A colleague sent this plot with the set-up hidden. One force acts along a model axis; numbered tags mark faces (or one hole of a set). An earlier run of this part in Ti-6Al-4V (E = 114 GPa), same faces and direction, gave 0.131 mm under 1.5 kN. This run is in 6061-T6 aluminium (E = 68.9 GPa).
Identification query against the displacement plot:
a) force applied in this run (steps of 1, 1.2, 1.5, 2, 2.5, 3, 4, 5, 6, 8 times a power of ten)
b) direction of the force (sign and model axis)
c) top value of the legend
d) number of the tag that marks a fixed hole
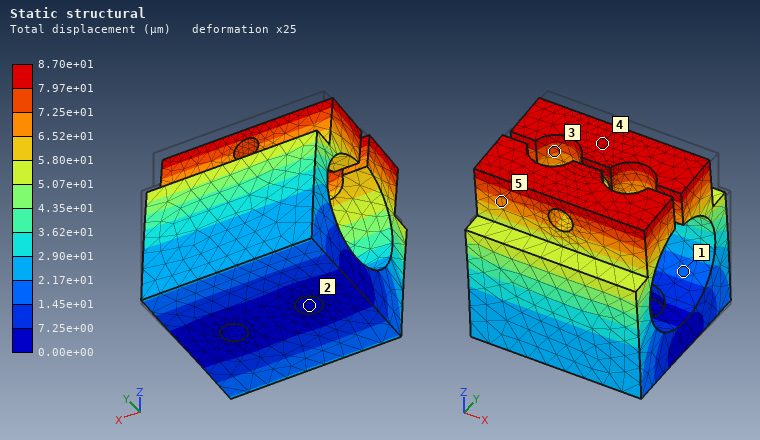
600 N
-Y
8.70e+01 µm
2
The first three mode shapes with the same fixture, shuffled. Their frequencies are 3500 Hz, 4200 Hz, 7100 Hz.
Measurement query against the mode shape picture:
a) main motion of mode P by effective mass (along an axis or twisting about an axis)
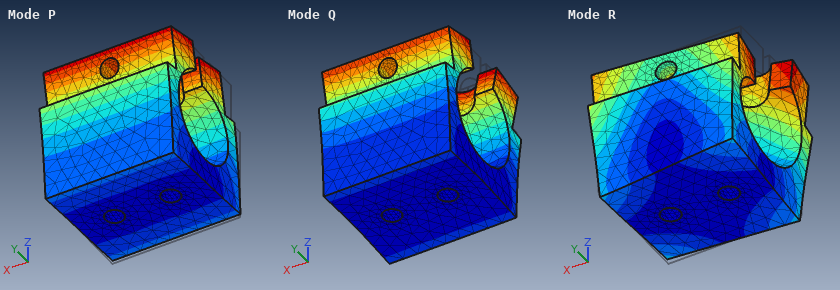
along Y
